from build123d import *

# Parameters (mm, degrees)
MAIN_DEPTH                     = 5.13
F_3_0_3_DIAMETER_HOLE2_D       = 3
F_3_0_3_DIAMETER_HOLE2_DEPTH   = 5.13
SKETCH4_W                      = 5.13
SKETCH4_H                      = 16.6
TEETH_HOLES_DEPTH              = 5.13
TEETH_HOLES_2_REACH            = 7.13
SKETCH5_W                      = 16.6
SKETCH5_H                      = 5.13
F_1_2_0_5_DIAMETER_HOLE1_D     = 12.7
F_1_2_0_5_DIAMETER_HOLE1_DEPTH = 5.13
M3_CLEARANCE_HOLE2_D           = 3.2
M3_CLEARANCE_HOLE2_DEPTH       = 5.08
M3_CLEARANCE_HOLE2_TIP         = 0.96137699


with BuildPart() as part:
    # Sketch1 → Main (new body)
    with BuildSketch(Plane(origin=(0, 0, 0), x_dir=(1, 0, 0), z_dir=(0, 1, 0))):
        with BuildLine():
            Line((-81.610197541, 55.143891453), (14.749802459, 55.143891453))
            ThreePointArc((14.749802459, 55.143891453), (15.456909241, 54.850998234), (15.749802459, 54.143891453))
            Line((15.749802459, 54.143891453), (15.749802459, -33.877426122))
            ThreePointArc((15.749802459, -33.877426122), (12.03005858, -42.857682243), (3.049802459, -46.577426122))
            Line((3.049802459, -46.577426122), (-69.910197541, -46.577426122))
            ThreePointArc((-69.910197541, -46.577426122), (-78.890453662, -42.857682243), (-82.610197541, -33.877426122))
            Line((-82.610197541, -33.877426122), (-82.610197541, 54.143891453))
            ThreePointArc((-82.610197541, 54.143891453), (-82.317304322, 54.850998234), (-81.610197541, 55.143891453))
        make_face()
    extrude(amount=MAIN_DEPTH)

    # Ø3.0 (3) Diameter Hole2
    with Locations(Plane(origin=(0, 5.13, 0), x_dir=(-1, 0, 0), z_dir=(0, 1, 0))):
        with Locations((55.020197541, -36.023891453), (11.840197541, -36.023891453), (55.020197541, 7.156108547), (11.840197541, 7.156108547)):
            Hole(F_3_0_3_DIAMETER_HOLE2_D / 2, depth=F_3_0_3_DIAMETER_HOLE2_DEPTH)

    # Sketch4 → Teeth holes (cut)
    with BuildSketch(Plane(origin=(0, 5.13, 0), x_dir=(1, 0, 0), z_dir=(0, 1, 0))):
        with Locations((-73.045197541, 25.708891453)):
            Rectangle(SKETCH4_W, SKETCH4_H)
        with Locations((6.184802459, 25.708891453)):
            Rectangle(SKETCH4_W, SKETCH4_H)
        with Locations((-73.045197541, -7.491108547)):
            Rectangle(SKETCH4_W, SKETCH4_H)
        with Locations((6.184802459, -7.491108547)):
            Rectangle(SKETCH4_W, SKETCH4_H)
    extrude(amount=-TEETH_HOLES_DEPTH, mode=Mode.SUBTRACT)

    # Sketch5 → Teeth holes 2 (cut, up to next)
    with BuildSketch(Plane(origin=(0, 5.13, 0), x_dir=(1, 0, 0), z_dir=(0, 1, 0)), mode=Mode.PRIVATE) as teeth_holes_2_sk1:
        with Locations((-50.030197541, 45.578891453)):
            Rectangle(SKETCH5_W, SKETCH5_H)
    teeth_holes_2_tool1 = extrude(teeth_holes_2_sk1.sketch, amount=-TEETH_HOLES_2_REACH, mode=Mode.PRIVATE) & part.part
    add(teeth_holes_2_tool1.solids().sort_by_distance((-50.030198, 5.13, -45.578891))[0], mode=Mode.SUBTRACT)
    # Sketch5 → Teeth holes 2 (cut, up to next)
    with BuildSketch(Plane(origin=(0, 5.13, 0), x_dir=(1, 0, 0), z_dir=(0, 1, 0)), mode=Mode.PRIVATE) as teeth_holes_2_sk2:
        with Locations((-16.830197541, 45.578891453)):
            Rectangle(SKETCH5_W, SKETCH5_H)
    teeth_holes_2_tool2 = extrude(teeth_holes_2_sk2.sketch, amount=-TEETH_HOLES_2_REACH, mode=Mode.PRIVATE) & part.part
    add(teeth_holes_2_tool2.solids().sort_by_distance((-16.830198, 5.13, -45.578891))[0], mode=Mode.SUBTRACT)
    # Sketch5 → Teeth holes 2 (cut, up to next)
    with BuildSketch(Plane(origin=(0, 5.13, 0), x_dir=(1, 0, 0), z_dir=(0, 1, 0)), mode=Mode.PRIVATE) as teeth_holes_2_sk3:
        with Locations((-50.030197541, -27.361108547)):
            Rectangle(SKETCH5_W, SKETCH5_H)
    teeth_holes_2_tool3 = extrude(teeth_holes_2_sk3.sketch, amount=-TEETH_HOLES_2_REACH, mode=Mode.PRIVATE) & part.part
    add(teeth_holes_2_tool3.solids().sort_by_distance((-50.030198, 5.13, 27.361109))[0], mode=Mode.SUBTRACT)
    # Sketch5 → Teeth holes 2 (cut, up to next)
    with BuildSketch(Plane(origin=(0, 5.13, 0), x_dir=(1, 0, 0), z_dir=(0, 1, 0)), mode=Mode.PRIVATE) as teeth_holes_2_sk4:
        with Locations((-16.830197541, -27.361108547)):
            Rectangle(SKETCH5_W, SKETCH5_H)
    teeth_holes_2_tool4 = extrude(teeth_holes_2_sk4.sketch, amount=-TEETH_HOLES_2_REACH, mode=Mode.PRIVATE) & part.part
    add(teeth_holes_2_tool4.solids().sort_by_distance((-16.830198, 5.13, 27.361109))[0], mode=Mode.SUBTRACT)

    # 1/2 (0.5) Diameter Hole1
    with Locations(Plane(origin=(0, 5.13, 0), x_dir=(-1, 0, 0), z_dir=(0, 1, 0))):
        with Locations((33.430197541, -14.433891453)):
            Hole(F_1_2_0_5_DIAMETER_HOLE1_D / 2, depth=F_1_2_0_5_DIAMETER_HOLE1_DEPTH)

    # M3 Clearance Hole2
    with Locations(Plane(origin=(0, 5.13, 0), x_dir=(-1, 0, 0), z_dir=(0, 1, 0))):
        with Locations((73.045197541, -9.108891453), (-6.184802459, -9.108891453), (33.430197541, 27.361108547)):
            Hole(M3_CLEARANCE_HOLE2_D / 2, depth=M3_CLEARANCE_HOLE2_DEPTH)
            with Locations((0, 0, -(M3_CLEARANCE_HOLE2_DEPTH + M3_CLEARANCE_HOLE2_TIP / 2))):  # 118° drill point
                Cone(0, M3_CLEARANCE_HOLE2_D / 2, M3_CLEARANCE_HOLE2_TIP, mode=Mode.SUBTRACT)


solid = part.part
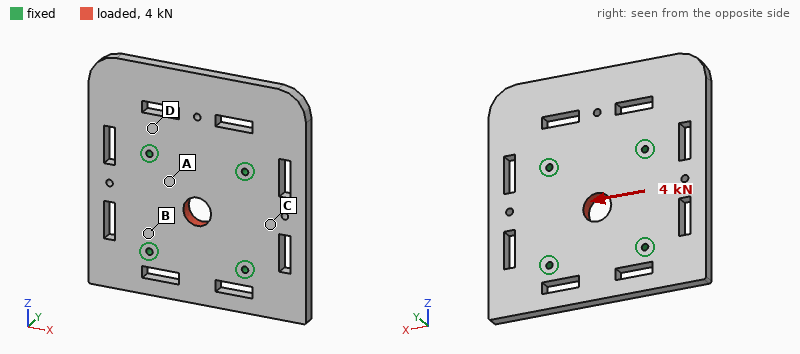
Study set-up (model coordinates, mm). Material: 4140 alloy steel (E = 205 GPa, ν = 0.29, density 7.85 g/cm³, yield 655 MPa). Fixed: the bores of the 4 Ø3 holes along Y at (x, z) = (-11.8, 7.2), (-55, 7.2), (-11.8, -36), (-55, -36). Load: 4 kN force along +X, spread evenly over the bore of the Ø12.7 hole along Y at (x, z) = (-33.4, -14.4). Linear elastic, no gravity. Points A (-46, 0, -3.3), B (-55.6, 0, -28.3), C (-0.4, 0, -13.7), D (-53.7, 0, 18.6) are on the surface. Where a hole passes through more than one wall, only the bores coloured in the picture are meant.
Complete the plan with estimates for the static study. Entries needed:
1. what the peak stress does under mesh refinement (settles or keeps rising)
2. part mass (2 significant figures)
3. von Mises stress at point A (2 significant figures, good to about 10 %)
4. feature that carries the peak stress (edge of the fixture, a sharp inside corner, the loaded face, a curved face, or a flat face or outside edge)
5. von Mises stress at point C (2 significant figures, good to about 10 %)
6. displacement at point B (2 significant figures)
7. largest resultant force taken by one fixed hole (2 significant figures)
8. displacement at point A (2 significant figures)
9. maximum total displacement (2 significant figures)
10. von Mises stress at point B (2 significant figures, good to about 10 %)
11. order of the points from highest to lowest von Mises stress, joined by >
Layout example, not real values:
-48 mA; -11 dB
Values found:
keeps rising; 370 g; 13 MPa; edge of the fixture; 5.5 MPa; 0.78 µm; 1.0 kN; 1.2 µm; 2.3 µm; 8.8 MPa; A > B > C > D
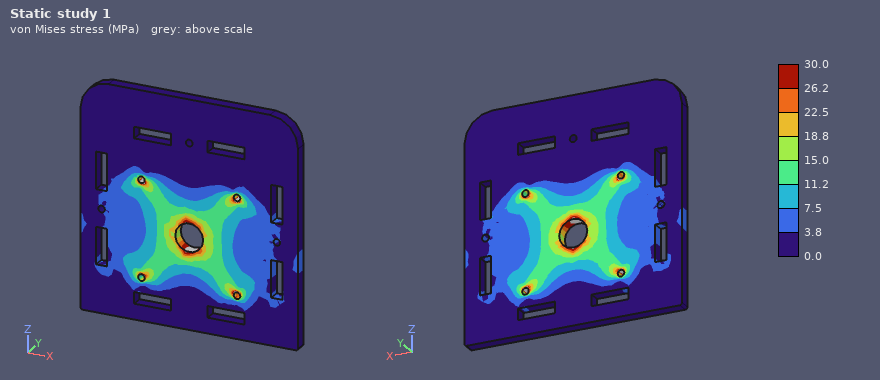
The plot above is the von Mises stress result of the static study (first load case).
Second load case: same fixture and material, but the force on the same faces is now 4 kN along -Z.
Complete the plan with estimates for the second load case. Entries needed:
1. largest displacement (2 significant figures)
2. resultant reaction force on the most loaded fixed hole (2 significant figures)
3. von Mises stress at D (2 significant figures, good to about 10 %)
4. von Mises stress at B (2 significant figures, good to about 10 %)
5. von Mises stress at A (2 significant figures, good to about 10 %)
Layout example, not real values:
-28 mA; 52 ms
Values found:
2.5 µm; 1.1 kN; 4.3 MPa; 9.1 MPa; 13 MPa
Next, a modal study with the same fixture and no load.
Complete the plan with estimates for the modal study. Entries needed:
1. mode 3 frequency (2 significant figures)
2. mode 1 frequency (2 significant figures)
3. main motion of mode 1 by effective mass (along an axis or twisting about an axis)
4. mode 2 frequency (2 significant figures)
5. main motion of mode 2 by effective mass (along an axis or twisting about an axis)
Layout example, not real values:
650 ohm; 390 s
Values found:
3900 Hz; 2100 Hz; along Y; 2700 Hz; twisting about Z
